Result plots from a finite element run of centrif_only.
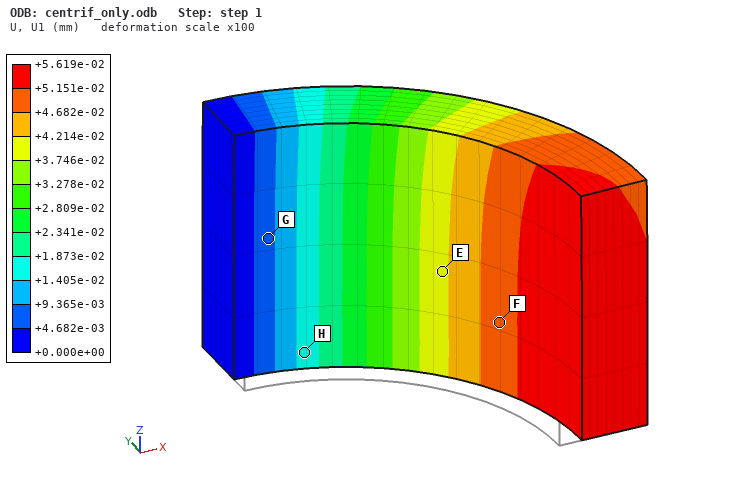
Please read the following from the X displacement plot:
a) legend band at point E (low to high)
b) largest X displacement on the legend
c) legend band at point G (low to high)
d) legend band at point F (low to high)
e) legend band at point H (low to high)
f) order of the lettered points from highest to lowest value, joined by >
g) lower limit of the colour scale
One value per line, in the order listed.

+3.746e-02 to +4.214e-02 mm
+5.619e-02 mm
+4.682e-03 to +9.365e-03 mm
+4.682e-02 to +5.151e-02 mm
+1.405e-02 to +1.873e-02 mm
F > E > H > G
+0.000e+00 mm
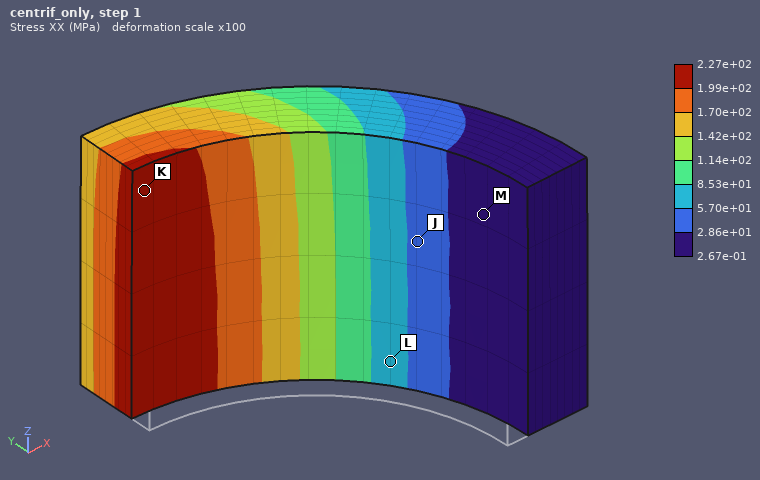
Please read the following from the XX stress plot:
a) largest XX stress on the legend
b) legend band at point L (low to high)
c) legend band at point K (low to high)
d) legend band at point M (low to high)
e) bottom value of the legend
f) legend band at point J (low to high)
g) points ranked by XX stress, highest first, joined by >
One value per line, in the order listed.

2.27e+02 MPa
5.70e+01 to 8.53e+01 MPa
1.99e+02 to 2.27e+02 MPa
2.67e-01 to 2.86e+01 MPa
2.67e-01 MPa
2.86e+01 to 5.70e+01 MPa
K > L > J > M
